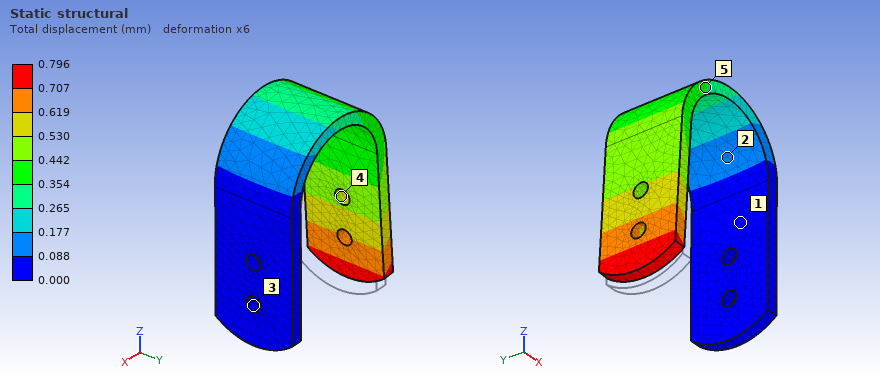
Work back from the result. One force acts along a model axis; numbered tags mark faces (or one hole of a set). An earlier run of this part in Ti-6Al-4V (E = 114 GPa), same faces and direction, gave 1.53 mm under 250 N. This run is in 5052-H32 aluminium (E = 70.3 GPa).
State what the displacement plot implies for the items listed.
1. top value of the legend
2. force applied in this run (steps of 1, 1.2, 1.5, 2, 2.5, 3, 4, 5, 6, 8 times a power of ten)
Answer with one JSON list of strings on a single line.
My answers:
["0.796 mm", "80 N"]
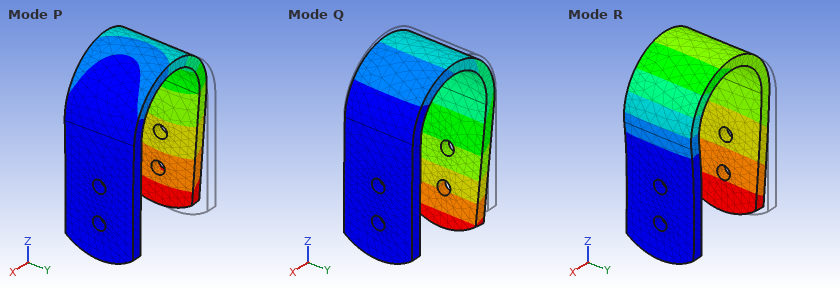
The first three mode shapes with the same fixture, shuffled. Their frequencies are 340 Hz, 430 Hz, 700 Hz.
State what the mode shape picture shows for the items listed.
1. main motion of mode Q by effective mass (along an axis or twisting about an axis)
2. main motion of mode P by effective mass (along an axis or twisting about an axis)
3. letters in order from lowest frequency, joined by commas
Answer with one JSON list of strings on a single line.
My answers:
["along Z", "along Y", "Q, P, R"]
